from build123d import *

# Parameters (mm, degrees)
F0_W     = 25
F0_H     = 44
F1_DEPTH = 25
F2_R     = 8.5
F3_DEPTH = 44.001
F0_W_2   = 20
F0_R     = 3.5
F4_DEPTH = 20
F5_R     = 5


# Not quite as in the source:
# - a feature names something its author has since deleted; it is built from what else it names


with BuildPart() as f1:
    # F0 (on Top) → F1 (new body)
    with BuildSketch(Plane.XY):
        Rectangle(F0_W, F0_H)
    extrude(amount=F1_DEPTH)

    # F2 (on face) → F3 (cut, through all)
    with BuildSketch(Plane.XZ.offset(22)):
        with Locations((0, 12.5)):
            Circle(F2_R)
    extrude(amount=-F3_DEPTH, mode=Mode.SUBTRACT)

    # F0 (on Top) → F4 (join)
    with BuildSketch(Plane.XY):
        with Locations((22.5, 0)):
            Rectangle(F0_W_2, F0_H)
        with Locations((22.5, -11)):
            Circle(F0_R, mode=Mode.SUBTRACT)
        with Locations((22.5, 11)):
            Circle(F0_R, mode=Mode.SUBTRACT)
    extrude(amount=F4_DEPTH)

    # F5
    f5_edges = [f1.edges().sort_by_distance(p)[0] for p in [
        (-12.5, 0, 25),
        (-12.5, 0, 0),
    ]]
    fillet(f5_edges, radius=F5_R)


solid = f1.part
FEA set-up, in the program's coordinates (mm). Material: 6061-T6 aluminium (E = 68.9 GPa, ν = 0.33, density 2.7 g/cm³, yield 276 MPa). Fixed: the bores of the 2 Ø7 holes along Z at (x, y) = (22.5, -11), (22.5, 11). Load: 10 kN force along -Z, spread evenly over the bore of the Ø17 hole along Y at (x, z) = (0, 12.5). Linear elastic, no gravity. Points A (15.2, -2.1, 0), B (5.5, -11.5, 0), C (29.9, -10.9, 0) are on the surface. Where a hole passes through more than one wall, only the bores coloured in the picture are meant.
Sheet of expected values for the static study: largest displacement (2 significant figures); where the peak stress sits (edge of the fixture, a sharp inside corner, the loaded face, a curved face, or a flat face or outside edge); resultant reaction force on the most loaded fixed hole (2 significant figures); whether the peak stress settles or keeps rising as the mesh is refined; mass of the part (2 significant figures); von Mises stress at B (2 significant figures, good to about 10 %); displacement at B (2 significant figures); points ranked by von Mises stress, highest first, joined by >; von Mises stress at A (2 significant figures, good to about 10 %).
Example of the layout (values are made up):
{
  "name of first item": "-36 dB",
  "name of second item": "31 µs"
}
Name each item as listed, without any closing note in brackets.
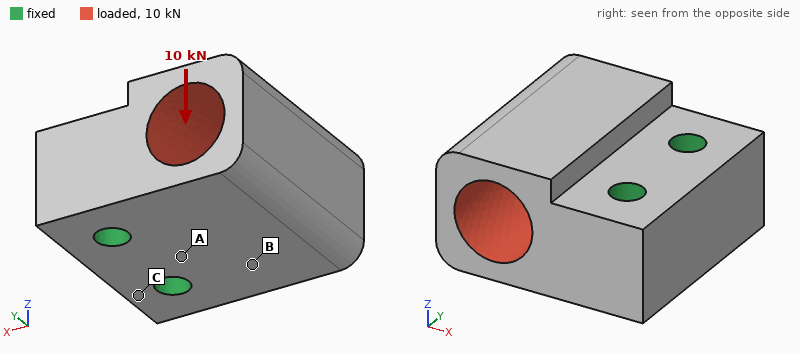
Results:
{
  "largest displacement": "98 µm",
  "where the peak stress sits": "edge of the fixture",
  "resultant reaction force on the most loaded fixed hole": "5.0 kN",
  "whether the peak stress settles or keeps rising as the mesh is refined": "keeps rising",
  "mass of the part": "89 g",
  "von Mises stress at B": "79 MPa",
  "displacement at B": "30 µm",
  "points ranked by von Mises stress, highest first, joined by >": "B > A > C",
  "von Mises stress at A": "42 MPa"
}
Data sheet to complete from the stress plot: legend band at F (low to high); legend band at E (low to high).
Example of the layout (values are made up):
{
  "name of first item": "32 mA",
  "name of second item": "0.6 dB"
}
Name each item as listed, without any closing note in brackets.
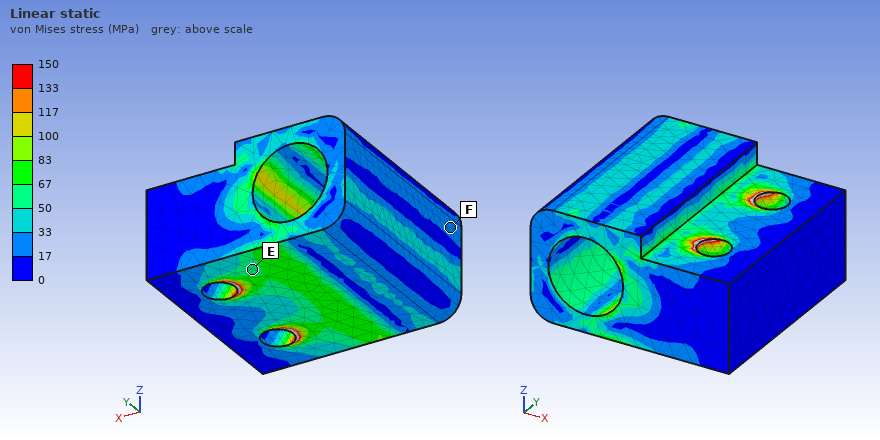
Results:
{
  "legend band at F": "17 to 33 MPa",
  "legend band at E": "50 to 67 MPa"
}
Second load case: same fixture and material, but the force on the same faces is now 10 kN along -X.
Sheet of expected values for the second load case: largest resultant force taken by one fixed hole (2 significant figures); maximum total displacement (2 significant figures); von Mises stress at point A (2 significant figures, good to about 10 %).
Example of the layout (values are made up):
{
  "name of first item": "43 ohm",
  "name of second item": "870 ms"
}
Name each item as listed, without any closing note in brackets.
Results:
{
  "largest resultant force taken by one fixed hole": "5.0 kN",
  "maximum total displacement": "23 µm",
  "von Mises stress at point A": "9.0 MPa"
}
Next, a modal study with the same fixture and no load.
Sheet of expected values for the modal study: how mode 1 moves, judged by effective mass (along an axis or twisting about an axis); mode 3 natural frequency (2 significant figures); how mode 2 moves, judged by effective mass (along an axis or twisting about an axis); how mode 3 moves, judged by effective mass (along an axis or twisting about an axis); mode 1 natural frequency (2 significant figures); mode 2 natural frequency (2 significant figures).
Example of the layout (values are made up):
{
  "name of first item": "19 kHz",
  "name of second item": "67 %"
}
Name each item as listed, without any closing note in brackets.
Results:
{
  "how mode 1 moves, judged by effective mass": "along Z",
  "mode 3 natural frequency": "16 kHz",
  "how mode 2 moves, judged by effective mass": "along Y",
  "how mode 3 moves, judged by effective mass": "twisting about X",
  "mode 1 natural frequency": "8400 Hz",
  "mode 2 natural frequency": "14 kHz"
}
